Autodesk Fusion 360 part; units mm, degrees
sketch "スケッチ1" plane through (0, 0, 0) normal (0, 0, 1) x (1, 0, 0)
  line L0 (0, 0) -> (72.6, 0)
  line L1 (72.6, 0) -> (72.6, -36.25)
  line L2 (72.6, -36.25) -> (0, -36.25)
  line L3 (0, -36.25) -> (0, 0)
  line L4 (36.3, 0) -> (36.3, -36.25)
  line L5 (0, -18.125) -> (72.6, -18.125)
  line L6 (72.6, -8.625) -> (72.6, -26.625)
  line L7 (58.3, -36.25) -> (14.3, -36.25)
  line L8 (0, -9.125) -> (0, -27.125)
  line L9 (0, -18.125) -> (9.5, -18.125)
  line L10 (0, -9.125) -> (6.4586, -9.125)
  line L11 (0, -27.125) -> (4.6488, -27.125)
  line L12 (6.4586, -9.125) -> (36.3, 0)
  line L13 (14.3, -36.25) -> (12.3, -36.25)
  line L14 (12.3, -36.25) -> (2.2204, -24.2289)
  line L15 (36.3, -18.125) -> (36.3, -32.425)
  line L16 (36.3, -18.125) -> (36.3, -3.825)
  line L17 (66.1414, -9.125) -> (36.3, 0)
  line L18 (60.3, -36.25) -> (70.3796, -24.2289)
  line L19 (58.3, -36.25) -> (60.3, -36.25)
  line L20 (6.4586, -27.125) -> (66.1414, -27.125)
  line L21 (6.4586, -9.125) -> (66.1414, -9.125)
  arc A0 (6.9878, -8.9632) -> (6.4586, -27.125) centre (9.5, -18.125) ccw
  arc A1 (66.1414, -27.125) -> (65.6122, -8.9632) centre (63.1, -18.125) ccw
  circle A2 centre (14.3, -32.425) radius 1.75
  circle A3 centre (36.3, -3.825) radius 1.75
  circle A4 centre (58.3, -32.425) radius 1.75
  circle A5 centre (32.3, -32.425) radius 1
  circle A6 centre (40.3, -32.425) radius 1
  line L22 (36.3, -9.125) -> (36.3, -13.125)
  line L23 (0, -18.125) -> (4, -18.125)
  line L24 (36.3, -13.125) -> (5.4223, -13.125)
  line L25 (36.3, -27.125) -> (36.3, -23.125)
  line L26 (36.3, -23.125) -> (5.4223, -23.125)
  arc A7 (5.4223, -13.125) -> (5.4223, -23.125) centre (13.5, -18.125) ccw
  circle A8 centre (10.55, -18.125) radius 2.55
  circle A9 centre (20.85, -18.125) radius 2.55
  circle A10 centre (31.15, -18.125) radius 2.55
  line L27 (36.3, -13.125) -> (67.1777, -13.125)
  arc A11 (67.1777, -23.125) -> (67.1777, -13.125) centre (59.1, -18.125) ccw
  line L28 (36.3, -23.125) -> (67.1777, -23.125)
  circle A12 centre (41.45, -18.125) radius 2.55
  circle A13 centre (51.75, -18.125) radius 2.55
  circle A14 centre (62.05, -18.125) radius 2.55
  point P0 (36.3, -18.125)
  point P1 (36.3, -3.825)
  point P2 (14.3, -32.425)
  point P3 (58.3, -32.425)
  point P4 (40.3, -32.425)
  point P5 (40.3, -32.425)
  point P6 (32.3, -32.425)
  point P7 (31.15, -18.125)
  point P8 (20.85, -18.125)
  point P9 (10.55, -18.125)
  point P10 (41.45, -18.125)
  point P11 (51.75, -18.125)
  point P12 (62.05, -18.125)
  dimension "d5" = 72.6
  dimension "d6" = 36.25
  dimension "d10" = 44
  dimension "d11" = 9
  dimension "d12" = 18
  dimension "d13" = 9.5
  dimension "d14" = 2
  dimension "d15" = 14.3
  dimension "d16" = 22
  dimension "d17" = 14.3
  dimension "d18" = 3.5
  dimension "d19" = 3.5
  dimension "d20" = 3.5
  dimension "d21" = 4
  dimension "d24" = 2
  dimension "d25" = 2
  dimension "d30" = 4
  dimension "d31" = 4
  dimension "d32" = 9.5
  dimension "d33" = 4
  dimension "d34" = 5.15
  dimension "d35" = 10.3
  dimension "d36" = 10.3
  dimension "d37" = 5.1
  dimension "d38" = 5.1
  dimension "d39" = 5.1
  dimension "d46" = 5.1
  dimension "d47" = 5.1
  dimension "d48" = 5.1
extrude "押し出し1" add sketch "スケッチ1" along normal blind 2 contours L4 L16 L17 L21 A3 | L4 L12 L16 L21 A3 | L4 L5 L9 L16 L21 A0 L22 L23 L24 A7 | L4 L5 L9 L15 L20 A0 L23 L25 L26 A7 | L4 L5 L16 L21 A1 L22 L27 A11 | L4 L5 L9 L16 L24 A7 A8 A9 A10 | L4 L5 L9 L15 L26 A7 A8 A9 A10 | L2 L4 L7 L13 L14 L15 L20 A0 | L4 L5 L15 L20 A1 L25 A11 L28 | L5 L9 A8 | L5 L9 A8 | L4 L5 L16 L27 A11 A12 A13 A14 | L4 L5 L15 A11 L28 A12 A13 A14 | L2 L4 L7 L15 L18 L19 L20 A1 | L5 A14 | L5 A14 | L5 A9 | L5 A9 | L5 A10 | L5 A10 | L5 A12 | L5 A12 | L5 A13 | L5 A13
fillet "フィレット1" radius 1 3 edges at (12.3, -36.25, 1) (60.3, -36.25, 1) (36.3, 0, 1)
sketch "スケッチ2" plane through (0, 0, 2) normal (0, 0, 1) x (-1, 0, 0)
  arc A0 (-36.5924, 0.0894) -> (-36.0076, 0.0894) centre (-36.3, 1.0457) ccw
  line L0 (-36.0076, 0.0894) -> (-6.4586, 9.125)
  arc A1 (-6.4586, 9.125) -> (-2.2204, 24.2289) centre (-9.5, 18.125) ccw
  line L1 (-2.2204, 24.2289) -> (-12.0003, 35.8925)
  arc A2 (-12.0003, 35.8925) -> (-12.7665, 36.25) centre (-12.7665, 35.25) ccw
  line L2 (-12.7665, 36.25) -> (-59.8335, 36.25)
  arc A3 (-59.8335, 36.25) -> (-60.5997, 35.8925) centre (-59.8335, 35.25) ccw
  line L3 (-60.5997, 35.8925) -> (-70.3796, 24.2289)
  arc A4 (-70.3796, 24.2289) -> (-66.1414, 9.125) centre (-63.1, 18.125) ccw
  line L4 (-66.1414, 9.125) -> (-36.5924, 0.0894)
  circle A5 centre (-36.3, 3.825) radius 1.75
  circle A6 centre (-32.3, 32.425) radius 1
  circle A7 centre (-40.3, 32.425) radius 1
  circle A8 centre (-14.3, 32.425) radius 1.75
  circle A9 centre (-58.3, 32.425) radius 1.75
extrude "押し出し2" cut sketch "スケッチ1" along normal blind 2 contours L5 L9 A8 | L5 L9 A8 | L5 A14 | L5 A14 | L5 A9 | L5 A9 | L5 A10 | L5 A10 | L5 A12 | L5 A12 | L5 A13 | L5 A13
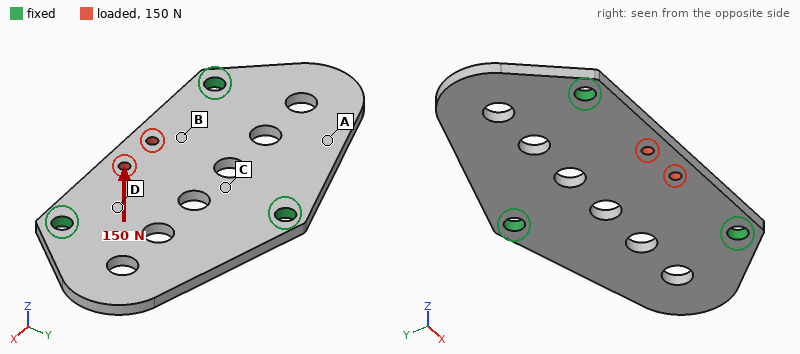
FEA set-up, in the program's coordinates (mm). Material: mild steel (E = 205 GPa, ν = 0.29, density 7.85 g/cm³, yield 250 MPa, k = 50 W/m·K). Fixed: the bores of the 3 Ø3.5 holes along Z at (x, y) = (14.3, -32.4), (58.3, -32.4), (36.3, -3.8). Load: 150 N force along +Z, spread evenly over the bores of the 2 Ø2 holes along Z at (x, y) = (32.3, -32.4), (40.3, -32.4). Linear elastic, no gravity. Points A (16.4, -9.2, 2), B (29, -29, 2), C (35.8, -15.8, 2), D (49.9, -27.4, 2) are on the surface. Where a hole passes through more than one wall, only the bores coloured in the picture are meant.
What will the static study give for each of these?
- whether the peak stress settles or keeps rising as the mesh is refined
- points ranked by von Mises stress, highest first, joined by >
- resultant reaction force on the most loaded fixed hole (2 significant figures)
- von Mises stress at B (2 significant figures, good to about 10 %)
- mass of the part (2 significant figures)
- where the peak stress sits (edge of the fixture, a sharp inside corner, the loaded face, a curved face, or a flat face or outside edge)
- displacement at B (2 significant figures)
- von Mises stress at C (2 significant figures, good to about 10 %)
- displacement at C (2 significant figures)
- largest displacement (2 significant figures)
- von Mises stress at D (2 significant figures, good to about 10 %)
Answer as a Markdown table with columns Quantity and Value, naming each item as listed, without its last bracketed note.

| Quantity | Value |
|---|---|
| whether the peak stress settles or keeps rising as the mesh is refined | keeps rising |
| points ranked by von Mises stress, highest first, joined by > | B > D > C > A |
| resultant reaction force on the most loaded fixed hole | 68 N |
| von Mises stress at B | 39 MPa |
| mass of the part | 29 g |
| where the peak stress sits | edge of the fixture |
| displacement at B | 18 µm |
| von Mises stress at C | 17 MPa |
| displacement at C | 6.3 µm |
| largest displacement | 35 µm |
| von Mises stress at D | 30 MPa |
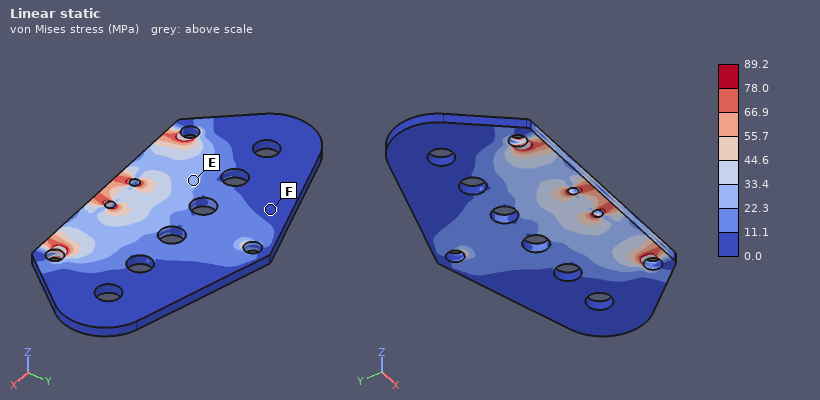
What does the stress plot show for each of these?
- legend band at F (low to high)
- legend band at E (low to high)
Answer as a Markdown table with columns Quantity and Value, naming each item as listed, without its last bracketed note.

| Quantity | Value |
|---|---|
| legend band at F | 0.0 to 11.1 MPa |
| legend band at E | 22.3 to 33.4 MPa |
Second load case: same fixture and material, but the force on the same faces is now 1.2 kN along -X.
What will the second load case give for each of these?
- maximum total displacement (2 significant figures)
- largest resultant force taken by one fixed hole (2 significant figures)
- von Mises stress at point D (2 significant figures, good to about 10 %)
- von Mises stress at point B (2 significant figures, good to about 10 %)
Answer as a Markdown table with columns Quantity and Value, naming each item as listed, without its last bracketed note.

| Quantity | Value |
|---|---|
| maximum total displacement | 3.1 µm |
| largest resultant force taken by one fixed hole | 530 N |
| von Mises stress at point D | 16 MPa |
| von Mises stress at point B | 22 MPa |
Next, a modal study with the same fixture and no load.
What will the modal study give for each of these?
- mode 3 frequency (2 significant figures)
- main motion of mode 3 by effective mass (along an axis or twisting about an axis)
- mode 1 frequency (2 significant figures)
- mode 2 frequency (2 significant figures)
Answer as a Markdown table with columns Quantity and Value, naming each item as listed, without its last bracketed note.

| Quantity | Value |
|---|---|
| mode 3 frequency | 6300 Hz |
| main motion of mode 3 by effective mass | along Z |
| mode 1 frequency | 3800 Hz |
| mode 2 frequency | 3800 Hz |
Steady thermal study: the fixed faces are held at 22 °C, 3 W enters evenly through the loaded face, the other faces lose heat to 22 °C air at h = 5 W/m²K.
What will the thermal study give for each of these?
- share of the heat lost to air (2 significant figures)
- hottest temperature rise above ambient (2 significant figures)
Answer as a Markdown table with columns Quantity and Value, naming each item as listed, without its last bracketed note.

| Quantity | Value |
|---|---|
| share of the heat lost to air | 3.4 % |
| hottest temperature rise above ambient | 19 K |
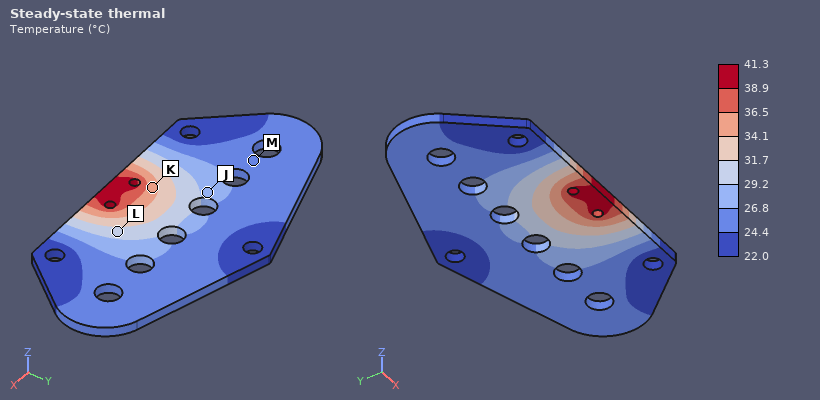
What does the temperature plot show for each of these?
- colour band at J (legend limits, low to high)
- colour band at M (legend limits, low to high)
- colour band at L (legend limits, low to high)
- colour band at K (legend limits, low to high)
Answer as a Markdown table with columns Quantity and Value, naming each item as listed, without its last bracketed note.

| Quantity | Value |
|---|---|
| colour band at J | 26.8 to 29.2 °C |
| colour band at M | 24.4 to 26.8 °C |
| colour band at L | 29.2 to 31.7 °C |
| colour band at K | 34.1 to 36.5 °C |
